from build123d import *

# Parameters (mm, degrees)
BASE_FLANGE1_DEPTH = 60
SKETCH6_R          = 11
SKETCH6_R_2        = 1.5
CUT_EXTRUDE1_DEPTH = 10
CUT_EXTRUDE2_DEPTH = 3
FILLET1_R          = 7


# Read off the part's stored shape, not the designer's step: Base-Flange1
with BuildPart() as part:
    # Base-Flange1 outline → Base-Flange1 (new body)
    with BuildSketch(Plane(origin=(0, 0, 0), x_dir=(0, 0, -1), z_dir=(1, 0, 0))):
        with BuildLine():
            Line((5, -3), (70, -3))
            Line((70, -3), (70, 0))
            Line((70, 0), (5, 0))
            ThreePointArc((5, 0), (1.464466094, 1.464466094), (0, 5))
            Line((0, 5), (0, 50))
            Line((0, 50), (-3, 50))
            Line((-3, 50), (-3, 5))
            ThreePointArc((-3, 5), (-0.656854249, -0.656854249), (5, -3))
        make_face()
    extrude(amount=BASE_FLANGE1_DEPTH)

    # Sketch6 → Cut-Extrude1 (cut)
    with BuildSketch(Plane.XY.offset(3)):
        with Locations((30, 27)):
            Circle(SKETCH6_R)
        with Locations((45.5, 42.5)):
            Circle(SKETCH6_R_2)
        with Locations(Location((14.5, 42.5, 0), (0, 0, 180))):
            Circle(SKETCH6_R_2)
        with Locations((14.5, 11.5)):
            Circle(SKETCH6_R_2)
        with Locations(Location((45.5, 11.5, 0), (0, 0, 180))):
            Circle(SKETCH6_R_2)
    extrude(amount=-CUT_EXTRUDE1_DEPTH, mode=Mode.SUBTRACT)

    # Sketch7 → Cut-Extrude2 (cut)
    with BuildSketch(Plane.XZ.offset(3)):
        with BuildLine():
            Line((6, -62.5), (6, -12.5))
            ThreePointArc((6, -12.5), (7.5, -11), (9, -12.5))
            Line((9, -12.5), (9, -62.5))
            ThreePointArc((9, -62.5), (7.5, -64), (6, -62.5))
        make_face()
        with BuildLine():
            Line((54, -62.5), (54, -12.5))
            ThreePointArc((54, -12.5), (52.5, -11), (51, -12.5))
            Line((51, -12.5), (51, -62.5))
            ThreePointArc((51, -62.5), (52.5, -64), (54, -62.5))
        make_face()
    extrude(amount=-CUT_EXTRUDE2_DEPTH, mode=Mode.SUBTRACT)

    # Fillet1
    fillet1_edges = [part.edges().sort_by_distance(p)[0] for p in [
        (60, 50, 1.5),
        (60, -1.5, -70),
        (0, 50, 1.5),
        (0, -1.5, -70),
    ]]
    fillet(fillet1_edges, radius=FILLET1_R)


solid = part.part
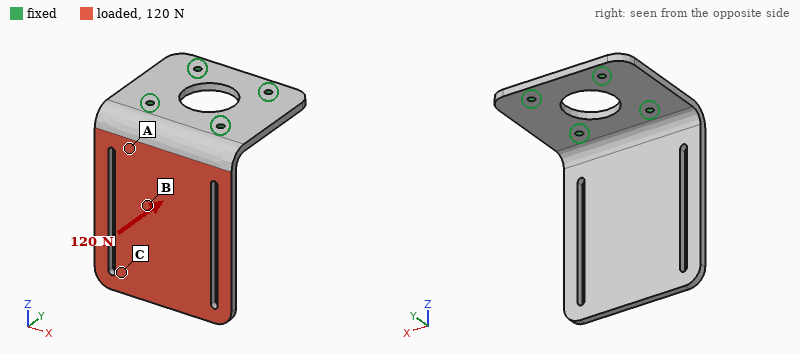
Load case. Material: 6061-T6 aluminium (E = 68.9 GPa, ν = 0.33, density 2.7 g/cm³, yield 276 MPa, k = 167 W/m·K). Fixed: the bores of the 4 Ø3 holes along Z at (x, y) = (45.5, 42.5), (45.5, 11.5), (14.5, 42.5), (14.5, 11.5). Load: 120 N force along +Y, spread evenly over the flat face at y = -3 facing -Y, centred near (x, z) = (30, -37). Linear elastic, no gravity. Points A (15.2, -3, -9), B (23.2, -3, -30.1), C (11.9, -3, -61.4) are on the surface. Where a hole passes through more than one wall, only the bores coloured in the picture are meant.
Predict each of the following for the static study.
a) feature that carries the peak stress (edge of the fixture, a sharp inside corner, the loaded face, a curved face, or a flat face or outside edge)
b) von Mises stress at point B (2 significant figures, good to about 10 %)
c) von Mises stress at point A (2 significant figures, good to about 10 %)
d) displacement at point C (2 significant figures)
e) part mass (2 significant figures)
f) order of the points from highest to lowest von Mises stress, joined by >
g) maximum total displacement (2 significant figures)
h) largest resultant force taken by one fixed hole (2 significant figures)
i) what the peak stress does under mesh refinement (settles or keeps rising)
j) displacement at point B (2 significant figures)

edge of the fixture
17 MPa
36 MPa
0.90 mm
52 g
A > B > C
1.1 mm
65 N
keeps rising
0.37 mm
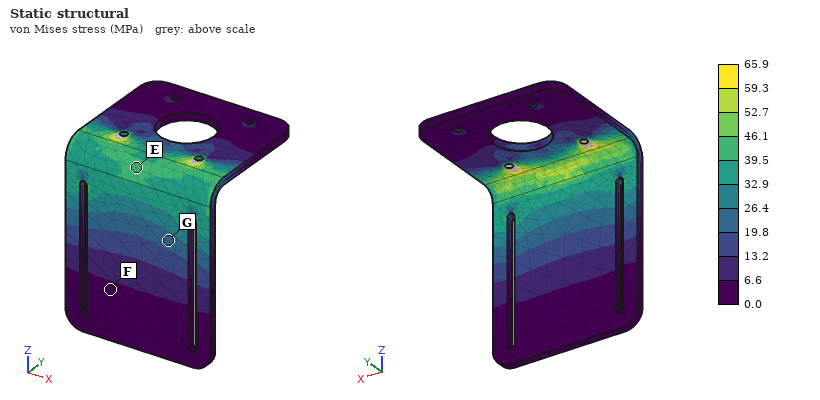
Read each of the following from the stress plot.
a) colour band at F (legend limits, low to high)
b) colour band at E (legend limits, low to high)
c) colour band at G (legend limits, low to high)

0.0 to 6.6 MPa
39.5 to 46.1 MPa
19.8 to 26.4 MPa
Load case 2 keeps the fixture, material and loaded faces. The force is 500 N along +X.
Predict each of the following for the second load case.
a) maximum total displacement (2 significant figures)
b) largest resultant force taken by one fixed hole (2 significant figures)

0.32 mm
670 N
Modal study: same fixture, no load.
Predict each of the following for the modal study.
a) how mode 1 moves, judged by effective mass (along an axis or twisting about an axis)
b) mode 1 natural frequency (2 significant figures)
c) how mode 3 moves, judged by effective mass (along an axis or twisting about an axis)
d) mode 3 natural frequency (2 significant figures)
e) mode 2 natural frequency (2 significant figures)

along Y
390 Hz
along X
1600 Hz
1100 Hz
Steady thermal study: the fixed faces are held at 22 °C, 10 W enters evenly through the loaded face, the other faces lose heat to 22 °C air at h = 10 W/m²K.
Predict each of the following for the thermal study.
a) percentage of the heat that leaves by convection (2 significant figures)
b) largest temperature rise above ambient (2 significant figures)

7.8 %
18 K
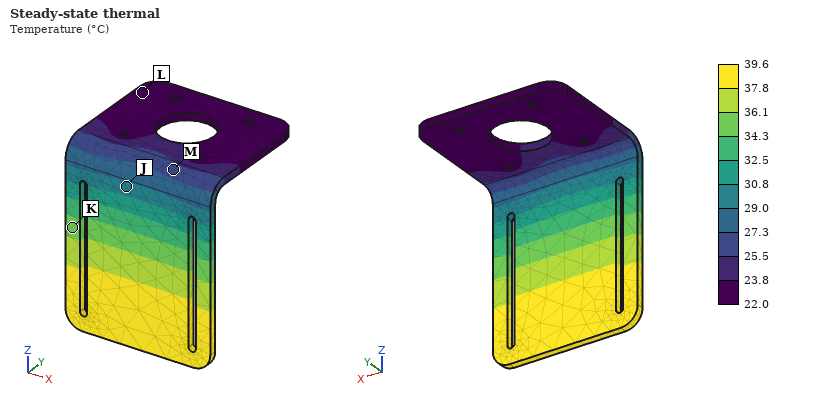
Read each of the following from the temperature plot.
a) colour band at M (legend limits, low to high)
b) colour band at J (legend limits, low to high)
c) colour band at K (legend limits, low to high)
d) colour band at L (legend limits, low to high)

25.5 to 27.3 °C
29.0 to 30.8 °C
34.3 to 36.1 °C
22.0 to 23.8 °C
